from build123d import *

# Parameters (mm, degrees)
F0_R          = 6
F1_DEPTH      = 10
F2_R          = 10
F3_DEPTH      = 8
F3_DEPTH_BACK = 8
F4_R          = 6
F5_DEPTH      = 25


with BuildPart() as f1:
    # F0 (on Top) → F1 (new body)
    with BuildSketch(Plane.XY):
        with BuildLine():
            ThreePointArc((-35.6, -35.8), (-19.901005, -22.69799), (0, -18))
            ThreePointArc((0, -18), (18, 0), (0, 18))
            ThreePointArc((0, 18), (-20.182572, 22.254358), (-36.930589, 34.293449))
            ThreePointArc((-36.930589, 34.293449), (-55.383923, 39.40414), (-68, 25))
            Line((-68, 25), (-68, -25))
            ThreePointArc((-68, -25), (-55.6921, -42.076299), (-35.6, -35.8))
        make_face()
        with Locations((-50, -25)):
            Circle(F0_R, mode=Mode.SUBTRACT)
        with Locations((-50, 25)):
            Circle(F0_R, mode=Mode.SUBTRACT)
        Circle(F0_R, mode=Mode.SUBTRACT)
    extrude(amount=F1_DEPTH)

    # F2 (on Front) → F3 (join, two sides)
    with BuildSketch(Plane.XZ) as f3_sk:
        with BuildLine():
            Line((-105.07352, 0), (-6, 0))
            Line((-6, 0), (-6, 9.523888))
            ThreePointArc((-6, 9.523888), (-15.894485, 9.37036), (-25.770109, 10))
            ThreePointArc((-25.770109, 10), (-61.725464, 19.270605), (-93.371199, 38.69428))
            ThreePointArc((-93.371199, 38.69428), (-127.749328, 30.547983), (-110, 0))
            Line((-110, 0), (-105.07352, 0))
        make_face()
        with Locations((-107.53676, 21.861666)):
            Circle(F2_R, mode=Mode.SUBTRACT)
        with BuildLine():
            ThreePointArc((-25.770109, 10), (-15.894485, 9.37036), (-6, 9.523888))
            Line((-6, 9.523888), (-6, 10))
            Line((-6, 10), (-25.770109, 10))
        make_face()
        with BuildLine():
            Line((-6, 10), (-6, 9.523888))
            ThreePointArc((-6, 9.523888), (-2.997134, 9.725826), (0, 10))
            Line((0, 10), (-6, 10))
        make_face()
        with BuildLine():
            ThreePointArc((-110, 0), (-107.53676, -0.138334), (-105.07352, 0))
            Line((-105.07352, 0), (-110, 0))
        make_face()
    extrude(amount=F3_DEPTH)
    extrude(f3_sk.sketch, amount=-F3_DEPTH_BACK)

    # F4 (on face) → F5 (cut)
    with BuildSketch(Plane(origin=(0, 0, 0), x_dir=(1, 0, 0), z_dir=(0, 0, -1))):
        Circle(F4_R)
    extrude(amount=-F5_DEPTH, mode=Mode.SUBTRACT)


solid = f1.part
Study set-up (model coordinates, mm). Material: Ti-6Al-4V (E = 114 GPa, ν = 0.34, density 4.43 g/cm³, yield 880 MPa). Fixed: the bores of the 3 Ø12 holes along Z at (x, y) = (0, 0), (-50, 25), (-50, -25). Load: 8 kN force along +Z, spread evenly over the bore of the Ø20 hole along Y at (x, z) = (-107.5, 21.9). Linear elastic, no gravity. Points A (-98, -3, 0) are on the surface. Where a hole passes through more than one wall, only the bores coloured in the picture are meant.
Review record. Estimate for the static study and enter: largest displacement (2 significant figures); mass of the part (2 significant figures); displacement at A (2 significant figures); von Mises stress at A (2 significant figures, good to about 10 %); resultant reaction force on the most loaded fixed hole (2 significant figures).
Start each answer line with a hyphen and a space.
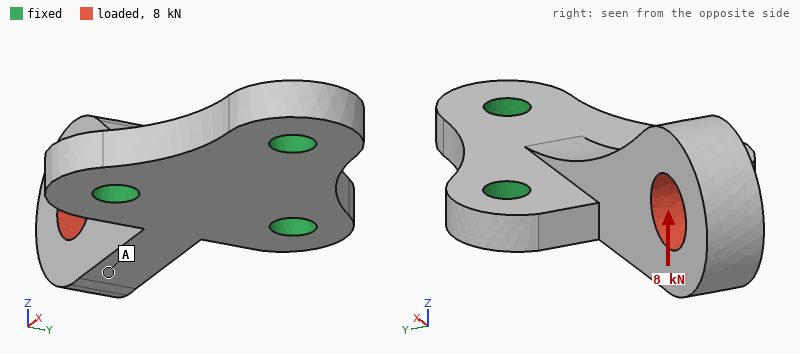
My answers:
- 0.95 mm
- 330 g
- 0.52 mm
- 55 MPa
- 7.6 kN
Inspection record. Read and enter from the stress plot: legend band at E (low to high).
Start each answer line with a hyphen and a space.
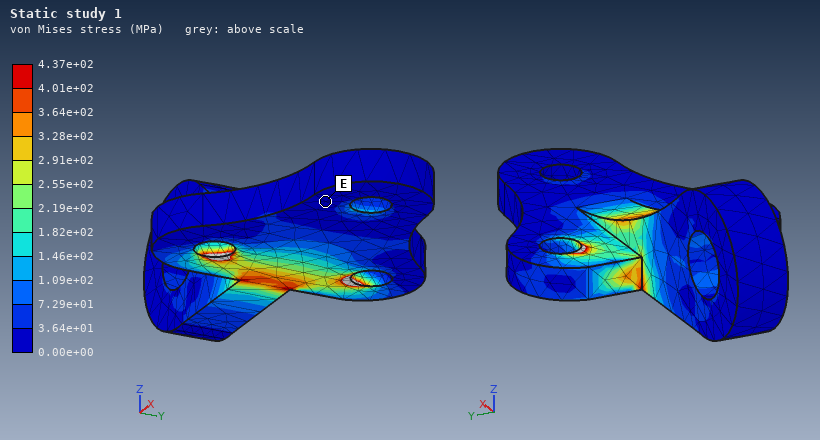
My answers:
- 0.00e+00 to 3.64e+01 MPa
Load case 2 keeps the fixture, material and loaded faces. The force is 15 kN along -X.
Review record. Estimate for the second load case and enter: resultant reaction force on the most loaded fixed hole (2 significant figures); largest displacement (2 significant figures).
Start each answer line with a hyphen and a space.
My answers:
- 5.3 kN
- 0.52 mm
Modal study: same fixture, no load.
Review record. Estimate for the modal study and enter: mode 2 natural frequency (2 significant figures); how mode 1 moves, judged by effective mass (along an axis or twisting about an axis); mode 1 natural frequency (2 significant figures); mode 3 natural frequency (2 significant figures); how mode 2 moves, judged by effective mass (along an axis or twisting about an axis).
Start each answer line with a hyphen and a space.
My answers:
- 2200 Hz
- along Z
- 1700 Hz
- 5500 Hz
- along Y
